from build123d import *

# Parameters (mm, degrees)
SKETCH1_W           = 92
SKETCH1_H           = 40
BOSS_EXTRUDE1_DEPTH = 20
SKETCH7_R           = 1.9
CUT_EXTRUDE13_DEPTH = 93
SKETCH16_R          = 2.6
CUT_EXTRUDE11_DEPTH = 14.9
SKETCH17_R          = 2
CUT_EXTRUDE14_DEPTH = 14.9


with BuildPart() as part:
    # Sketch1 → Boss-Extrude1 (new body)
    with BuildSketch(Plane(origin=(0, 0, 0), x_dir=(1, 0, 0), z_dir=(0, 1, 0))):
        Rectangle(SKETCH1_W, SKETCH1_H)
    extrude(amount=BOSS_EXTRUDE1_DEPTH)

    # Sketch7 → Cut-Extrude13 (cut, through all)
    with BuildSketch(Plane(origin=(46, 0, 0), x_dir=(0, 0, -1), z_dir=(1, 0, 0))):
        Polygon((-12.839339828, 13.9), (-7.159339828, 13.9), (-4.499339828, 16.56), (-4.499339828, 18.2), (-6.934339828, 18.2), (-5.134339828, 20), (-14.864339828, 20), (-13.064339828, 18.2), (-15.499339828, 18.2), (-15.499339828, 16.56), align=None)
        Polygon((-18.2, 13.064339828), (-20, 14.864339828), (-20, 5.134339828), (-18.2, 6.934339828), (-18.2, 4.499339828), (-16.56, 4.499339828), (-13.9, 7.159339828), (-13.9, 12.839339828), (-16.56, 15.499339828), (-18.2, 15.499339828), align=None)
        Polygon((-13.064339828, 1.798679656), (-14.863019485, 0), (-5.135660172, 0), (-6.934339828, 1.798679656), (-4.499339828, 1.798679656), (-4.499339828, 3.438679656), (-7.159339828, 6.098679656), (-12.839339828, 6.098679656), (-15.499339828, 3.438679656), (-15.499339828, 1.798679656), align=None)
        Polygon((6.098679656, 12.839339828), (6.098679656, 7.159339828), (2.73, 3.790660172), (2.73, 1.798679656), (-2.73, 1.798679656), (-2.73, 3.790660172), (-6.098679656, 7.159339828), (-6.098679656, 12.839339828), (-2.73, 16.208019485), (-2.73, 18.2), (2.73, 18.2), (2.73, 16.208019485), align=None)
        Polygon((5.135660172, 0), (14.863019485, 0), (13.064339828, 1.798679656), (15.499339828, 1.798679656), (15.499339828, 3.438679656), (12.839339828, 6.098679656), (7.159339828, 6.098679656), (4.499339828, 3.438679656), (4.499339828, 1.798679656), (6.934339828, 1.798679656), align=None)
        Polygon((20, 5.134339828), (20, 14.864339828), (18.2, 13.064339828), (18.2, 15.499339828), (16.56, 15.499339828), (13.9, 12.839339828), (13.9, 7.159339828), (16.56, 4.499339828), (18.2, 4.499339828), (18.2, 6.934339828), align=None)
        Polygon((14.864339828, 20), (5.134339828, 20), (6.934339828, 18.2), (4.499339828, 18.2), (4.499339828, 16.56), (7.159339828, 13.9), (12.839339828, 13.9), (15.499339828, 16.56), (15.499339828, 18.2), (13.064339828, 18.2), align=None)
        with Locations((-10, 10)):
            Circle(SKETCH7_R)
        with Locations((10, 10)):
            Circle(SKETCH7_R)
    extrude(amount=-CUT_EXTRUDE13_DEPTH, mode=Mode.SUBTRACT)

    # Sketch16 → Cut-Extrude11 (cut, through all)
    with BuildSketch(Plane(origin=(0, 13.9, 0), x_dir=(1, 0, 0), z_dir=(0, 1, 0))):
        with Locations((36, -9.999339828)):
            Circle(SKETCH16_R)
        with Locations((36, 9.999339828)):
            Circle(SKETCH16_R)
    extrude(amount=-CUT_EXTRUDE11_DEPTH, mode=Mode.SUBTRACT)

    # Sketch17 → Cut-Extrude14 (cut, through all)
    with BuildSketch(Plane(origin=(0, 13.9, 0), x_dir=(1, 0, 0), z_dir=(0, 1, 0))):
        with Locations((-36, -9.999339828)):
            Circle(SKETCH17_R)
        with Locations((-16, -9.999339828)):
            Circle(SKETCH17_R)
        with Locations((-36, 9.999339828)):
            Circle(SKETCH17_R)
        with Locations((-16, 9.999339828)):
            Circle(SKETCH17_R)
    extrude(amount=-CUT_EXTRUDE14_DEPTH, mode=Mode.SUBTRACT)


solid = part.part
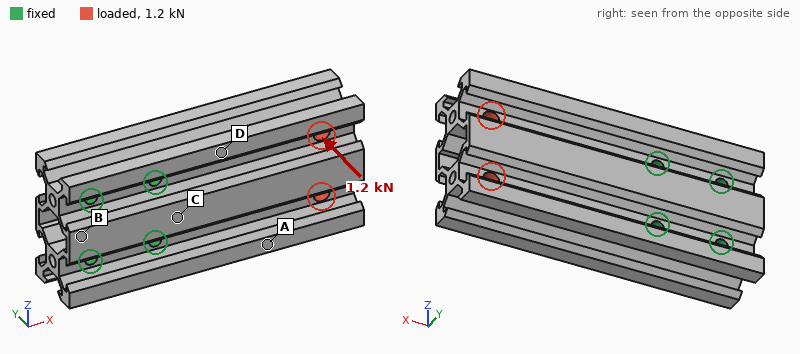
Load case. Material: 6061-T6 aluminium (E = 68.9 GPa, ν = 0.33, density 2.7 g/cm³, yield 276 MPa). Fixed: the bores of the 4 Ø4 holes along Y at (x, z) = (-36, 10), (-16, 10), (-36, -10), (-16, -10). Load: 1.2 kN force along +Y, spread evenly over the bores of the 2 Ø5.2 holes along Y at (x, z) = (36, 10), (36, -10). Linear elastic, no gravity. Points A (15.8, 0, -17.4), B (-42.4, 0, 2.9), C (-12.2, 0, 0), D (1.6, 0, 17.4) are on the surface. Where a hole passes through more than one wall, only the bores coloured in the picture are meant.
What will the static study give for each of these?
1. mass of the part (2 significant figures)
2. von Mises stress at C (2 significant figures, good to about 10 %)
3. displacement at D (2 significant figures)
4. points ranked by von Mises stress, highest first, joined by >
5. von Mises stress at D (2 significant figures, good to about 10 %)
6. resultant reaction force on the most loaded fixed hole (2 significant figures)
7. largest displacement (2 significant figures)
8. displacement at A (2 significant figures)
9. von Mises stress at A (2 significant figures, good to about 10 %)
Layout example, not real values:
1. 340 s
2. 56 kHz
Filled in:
1. 73 g
2. 49 MPa
3. 0.042 mm
4. C > D > A > B
5. 35 MPa
6. 1.5 kN
7. 0.18 mm
8. 0.081 mm
9. 20 MPa
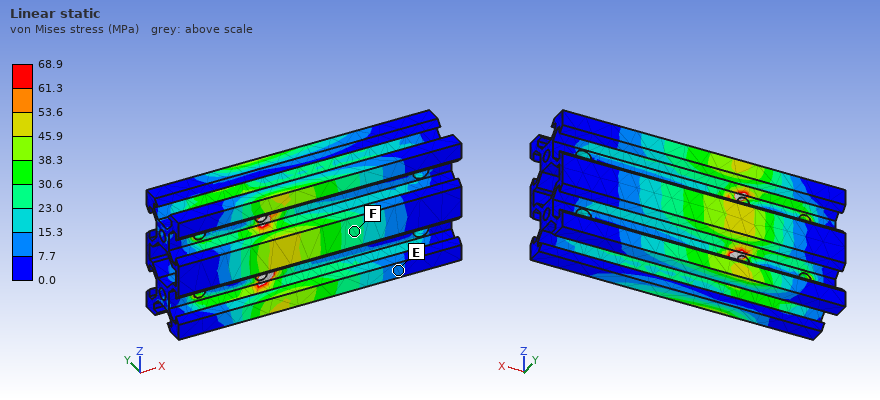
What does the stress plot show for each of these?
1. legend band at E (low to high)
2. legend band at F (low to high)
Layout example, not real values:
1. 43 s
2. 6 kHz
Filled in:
1. 7.7 to 15.3 MPa
2. 23.0 to 30.6 MPa
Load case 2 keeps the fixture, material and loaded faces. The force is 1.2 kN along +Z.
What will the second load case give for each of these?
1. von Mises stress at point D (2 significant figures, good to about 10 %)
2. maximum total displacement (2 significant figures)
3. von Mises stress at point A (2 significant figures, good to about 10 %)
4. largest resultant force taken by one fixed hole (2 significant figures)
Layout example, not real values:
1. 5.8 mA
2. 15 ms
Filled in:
1. 13 MPa
2. 65 µm
3. 8.7 MPa
4. 1.8 kN
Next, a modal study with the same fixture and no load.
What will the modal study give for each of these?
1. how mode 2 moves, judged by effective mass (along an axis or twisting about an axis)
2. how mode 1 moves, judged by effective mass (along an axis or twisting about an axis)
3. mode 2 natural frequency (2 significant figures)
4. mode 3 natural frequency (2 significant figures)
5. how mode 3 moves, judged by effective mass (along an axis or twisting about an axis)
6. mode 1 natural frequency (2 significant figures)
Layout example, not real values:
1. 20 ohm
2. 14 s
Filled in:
1. twisting about X
2. along Y
3. 4300 Hz
4. 4800 Hz
5. along Z
6. 3000 Hz
